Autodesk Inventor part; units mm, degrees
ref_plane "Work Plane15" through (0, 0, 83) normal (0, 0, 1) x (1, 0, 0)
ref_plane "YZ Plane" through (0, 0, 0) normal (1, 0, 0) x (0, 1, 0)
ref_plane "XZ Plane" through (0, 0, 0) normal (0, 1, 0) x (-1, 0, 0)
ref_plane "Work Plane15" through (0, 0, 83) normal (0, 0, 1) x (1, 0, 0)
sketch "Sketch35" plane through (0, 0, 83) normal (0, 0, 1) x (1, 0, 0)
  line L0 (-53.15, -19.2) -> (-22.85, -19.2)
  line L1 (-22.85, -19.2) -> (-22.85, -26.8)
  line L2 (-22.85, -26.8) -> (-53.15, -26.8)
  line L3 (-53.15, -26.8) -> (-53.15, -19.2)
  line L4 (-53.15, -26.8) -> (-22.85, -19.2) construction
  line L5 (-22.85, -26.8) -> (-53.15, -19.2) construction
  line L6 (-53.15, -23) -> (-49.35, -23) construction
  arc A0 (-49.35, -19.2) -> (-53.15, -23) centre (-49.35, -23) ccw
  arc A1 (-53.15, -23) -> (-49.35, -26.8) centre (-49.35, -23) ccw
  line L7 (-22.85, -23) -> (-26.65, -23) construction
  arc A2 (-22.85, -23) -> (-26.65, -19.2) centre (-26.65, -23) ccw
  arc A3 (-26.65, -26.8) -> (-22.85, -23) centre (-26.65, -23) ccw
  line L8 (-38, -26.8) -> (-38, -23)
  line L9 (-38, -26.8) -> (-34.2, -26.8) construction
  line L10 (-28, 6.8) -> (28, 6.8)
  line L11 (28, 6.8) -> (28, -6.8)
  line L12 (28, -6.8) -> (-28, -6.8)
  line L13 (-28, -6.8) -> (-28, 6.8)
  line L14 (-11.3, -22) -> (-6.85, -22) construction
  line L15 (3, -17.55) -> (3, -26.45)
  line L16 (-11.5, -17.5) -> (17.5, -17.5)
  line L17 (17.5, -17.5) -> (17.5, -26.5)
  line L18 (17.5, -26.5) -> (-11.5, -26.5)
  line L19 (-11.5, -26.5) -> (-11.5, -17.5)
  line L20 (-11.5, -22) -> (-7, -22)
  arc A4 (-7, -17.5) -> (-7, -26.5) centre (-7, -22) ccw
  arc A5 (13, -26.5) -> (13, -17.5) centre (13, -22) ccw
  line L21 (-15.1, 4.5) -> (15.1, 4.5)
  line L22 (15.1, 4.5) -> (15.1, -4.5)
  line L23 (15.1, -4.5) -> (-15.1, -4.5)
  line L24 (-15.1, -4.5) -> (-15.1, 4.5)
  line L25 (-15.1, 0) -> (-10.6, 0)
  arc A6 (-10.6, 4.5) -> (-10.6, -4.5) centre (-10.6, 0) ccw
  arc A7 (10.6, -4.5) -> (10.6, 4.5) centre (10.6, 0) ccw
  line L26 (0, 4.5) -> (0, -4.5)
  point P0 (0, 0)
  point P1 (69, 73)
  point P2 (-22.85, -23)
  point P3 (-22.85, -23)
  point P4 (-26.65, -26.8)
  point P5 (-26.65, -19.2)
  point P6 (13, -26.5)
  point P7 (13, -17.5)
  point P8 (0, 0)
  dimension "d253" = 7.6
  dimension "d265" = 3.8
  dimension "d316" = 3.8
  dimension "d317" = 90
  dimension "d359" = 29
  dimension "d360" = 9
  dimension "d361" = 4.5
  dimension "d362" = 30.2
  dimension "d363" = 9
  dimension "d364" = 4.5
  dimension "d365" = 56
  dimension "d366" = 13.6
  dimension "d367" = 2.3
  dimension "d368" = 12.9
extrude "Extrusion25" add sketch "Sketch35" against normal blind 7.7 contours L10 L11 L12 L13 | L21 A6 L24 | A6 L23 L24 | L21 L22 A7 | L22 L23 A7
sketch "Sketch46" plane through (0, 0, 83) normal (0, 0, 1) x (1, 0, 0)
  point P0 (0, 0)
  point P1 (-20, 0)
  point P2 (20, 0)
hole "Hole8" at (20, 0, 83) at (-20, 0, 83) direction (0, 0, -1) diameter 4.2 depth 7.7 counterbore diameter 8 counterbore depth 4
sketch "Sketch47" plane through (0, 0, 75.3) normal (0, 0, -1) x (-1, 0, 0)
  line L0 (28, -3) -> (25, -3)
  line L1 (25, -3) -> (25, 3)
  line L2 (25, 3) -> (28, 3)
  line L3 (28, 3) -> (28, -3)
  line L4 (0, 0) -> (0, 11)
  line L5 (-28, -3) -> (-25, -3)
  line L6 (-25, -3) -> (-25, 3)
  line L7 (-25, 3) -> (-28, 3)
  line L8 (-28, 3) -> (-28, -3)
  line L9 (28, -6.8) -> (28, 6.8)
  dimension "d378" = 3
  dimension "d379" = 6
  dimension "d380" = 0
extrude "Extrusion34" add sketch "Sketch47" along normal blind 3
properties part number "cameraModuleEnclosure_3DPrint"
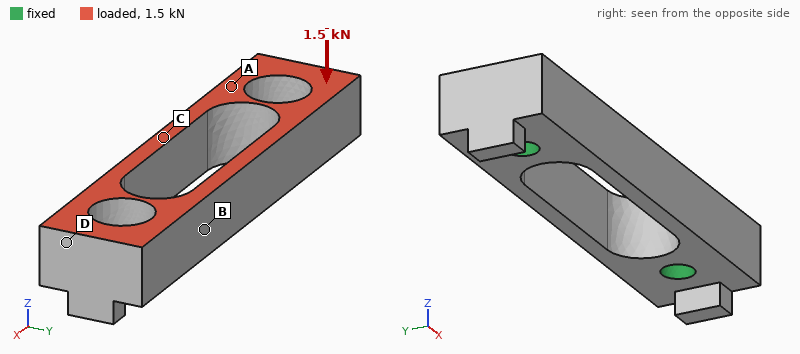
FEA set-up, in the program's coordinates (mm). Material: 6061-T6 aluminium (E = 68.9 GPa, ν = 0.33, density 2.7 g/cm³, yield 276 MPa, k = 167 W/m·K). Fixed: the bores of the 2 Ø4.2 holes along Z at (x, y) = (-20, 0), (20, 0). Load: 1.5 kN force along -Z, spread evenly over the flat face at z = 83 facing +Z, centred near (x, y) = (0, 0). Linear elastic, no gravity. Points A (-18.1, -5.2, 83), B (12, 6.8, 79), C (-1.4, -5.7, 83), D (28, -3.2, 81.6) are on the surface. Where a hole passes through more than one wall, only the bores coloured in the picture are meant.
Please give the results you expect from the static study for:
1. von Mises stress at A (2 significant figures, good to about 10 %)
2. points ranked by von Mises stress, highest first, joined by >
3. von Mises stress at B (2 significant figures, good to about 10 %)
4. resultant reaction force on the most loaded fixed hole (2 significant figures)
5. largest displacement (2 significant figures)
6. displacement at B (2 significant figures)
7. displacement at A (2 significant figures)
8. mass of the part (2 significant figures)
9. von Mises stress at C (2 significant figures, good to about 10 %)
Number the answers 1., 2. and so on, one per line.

1. 19 MPa
2. C > A > B > D
3. 14 MPa
4. 760 N
5. 15 µm
6. 7.5 µm
7. 3.8 µm
8. 9.5 g
9. 26 MPa
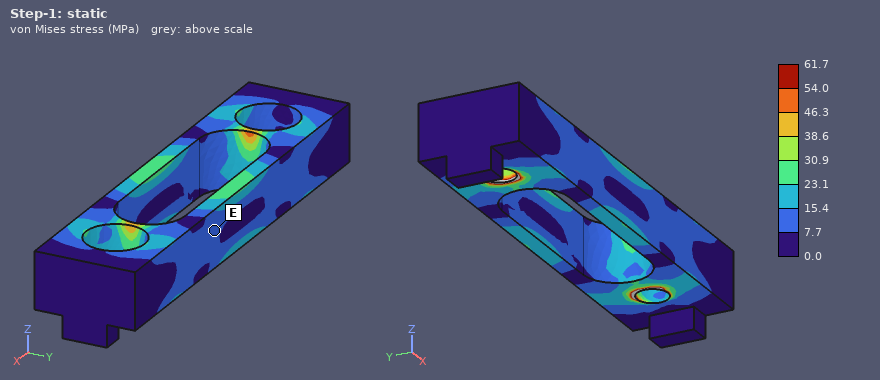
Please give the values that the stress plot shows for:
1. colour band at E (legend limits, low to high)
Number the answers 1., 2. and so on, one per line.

1. 7.7 to 15.4 MPa
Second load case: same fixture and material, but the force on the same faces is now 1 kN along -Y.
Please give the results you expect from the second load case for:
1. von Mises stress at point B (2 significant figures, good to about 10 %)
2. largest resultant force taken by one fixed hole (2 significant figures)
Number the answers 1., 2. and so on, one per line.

1. 30 MPa
2. 500 N
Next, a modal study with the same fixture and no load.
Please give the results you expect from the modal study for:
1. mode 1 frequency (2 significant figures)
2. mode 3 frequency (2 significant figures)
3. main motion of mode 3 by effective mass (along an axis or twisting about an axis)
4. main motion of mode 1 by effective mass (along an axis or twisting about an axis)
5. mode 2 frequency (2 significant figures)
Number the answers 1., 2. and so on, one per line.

1. 14 kHz
2. 19 kHz
3. along Z
4. along Y
5. 14 kHz
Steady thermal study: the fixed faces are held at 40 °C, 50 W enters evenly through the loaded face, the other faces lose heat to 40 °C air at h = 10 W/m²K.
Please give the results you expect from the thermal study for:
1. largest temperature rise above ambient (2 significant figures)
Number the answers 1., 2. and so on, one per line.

1. 21 K
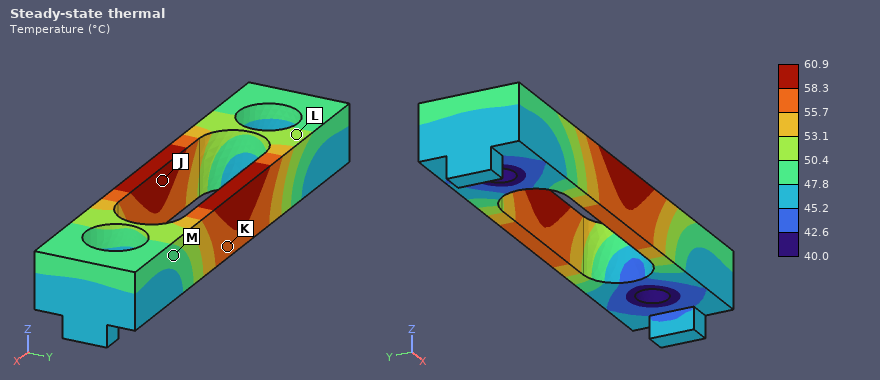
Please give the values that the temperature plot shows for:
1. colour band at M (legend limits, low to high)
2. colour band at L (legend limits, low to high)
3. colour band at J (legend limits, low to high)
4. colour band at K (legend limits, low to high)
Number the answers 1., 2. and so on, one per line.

1. 47.8 to 50.4 °C
2. 50.4 to 53.1 °C
3. 58.3 to 60.9 °C
4. 55.7 to 58.3 °C
